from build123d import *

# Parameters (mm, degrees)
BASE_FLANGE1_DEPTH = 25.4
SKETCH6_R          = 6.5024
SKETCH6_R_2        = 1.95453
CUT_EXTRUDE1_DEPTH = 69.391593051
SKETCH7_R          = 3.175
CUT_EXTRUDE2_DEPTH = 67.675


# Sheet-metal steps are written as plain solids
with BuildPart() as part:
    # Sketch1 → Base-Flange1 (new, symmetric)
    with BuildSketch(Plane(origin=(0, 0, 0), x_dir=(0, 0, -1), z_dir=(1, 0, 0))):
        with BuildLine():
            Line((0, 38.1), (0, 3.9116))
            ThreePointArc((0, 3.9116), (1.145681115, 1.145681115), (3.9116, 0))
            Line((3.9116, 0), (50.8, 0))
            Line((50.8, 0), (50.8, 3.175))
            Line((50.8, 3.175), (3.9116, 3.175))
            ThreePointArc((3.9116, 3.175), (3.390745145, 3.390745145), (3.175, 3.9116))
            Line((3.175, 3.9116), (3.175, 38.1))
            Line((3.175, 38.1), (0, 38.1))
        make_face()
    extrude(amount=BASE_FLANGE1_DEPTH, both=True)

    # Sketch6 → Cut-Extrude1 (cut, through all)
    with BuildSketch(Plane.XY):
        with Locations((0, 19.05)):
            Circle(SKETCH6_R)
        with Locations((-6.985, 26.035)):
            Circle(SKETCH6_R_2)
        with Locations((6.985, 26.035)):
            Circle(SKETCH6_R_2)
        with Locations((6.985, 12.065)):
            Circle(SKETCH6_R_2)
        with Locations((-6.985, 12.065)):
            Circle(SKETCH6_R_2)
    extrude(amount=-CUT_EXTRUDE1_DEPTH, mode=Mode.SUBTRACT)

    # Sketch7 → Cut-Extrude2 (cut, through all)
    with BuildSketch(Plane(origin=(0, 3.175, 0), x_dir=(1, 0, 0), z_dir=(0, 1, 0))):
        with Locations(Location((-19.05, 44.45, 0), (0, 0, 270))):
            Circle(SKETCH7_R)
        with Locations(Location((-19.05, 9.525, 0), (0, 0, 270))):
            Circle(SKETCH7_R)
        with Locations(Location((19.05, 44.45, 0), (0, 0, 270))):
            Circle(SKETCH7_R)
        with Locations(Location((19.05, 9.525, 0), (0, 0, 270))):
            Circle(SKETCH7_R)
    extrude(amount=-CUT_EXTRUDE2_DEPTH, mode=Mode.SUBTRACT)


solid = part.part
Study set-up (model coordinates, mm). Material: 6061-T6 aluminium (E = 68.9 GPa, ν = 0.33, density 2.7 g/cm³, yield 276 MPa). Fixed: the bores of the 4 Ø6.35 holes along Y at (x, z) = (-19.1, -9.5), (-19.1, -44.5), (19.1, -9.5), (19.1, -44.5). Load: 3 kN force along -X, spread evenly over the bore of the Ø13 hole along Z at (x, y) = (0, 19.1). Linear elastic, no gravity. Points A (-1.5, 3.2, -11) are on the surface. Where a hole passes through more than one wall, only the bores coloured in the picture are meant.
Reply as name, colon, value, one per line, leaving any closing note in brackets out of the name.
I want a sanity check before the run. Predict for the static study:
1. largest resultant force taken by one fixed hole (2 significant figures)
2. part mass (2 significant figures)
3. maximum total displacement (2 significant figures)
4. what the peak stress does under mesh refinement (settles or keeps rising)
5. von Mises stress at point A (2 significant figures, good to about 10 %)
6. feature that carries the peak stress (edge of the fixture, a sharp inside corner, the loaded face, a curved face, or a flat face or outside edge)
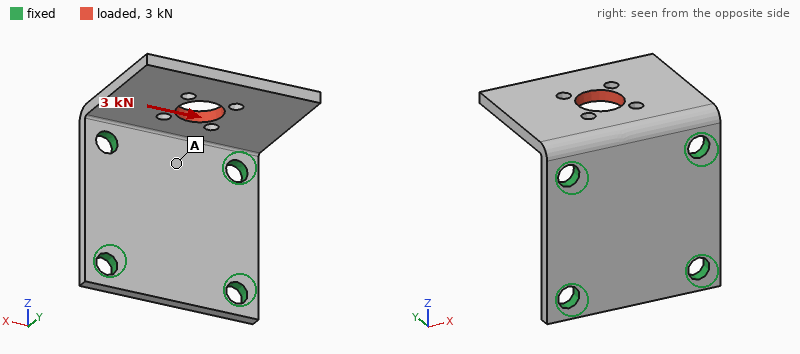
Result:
largest resultant force taken by one fixed hole: 2.0 kN
part mass: 34 g
maximum total displacement: 0.15 mm
what the peak stress does under mesh refinement: keeps rising
von Mises stress at point A: 23 MPa
feature that carries the peak stress: edge of the fixture
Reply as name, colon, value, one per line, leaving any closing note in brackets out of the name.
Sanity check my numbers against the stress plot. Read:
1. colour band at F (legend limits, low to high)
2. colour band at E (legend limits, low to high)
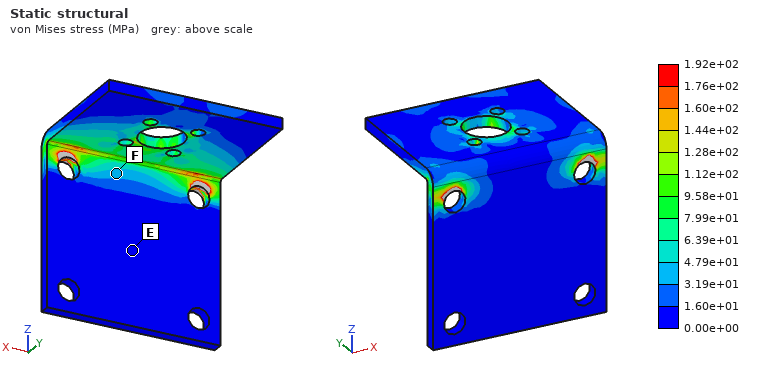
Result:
colour band at F: 3.19e+01 to 4.79e+01 MPa
colour band at E: 0.00e+00 to 1.60e+01 MPa
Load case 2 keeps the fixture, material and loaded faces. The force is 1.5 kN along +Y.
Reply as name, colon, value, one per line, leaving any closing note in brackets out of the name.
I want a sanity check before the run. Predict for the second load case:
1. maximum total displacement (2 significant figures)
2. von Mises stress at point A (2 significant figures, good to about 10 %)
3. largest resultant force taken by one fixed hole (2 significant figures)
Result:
maximum total displacement: 0.14 mm
von Mises stress at point A: 22 MPa
largest resultant force taken by one fixed hole: 790 N
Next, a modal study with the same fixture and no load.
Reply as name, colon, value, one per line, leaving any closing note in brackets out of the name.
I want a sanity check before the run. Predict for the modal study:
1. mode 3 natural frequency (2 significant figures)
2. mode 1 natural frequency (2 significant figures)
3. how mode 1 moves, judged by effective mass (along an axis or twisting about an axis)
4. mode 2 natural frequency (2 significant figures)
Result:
mode 3 natural frequency: 8000 Hz
mode 1 natural frequency: 1500 Hz
how mode 1 moves, judged by effective mass: along Z
mode 2 natural frequency: 3100 Hz
